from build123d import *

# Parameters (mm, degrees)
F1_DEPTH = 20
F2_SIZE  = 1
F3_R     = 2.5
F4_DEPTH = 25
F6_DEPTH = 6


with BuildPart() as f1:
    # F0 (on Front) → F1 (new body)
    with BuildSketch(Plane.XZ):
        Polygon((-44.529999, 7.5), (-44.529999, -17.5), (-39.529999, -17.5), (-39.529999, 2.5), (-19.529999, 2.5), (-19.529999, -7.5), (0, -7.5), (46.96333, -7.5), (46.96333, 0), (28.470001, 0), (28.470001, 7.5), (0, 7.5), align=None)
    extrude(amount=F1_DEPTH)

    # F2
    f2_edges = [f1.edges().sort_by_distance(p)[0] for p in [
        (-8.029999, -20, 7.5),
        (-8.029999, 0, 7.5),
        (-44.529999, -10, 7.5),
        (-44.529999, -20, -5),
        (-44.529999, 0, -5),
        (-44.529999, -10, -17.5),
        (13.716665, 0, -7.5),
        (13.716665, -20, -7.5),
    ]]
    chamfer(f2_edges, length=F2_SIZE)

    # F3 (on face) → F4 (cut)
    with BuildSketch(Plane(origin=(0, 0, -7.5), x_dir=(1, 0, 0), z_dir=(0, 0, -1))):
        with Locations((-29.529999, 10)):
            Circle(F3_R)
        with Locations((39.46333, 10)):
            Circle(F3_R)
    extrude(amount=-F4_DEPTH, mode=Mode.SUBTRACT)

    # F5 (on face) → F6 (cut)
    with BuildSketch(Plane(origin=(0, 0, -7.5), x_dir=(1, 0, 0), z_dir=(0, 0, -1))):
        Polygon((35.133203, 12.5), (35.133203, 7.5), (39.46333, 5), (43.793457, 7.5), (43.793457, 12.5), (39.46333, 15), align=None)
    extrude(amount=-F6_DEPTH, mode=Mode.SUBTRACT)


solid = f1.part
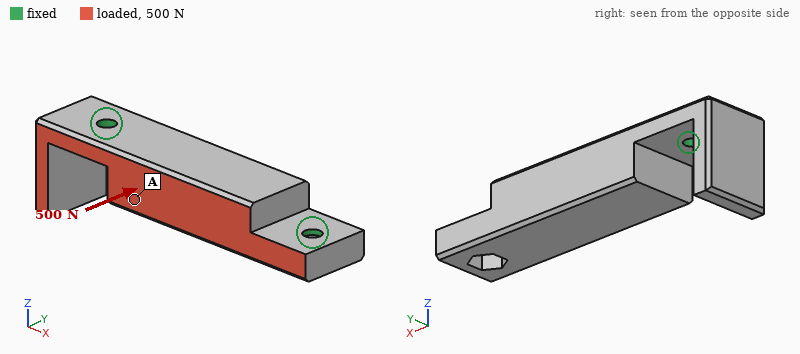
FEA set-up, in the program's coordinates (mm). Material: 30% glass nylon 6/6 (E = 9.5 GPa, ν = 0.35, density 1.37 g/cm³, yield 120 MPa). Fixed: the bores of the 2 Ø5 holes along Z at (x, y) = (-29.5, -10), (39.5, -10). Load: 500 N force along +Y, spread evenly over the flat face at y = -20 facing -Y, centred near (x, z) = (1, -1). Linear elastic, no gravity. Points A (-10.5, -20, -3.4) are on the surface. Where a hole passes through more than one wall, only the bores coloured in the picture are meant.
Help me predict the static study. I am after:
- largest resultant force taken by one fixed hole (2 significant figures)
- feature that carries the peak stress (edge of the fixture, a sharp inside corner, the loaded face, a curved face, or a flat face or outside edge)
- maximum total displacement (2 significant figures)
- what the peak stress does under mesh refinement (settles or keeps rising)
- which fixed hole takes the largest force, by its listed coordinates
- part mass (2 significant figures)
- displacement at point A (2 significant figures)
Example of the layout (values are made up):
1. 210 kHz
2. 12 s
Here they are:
1. 280 N
2. edge of the fixture
3. 53 µm
4. keeps rising
5. (-29.5, -10)
6. 29 g
7. 44 µm
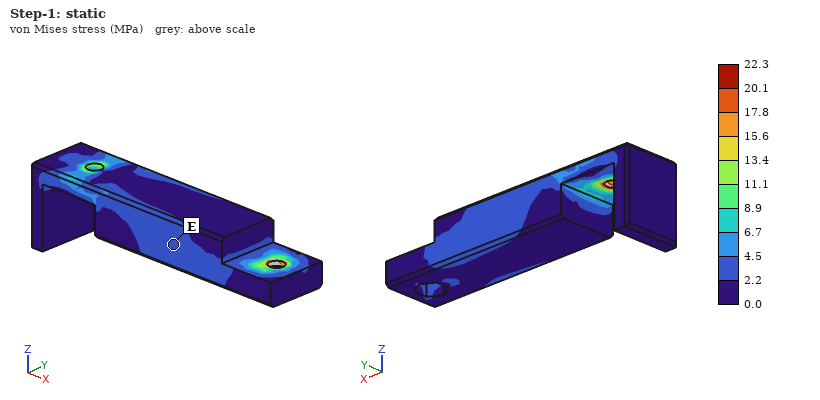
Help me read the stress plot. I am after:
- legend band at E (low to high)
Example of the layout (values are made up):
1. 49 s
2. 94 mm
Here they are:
1. 2.2 to 4.5 MPa
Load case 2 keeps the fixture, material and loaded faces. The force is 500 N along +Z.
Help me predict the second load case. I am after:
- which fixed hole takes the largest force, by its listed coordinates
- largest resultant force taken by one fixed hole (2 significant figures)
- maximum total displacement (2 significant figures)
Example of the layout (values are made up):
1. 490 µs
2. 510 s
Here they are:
1. (-29.5, -10)
2. 330 N
3. 0.17 mm
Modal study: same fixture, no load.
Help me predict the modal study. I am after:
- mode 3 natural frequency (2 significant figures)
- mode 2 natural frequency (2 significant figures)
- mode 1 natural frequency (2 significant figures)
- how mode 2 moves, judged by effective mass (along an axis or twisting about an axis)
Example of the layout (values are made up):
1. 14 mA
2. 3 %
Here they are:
1. 3200 Hz
2. 2800 Hz
3. 2300 Hz
4. along Y
